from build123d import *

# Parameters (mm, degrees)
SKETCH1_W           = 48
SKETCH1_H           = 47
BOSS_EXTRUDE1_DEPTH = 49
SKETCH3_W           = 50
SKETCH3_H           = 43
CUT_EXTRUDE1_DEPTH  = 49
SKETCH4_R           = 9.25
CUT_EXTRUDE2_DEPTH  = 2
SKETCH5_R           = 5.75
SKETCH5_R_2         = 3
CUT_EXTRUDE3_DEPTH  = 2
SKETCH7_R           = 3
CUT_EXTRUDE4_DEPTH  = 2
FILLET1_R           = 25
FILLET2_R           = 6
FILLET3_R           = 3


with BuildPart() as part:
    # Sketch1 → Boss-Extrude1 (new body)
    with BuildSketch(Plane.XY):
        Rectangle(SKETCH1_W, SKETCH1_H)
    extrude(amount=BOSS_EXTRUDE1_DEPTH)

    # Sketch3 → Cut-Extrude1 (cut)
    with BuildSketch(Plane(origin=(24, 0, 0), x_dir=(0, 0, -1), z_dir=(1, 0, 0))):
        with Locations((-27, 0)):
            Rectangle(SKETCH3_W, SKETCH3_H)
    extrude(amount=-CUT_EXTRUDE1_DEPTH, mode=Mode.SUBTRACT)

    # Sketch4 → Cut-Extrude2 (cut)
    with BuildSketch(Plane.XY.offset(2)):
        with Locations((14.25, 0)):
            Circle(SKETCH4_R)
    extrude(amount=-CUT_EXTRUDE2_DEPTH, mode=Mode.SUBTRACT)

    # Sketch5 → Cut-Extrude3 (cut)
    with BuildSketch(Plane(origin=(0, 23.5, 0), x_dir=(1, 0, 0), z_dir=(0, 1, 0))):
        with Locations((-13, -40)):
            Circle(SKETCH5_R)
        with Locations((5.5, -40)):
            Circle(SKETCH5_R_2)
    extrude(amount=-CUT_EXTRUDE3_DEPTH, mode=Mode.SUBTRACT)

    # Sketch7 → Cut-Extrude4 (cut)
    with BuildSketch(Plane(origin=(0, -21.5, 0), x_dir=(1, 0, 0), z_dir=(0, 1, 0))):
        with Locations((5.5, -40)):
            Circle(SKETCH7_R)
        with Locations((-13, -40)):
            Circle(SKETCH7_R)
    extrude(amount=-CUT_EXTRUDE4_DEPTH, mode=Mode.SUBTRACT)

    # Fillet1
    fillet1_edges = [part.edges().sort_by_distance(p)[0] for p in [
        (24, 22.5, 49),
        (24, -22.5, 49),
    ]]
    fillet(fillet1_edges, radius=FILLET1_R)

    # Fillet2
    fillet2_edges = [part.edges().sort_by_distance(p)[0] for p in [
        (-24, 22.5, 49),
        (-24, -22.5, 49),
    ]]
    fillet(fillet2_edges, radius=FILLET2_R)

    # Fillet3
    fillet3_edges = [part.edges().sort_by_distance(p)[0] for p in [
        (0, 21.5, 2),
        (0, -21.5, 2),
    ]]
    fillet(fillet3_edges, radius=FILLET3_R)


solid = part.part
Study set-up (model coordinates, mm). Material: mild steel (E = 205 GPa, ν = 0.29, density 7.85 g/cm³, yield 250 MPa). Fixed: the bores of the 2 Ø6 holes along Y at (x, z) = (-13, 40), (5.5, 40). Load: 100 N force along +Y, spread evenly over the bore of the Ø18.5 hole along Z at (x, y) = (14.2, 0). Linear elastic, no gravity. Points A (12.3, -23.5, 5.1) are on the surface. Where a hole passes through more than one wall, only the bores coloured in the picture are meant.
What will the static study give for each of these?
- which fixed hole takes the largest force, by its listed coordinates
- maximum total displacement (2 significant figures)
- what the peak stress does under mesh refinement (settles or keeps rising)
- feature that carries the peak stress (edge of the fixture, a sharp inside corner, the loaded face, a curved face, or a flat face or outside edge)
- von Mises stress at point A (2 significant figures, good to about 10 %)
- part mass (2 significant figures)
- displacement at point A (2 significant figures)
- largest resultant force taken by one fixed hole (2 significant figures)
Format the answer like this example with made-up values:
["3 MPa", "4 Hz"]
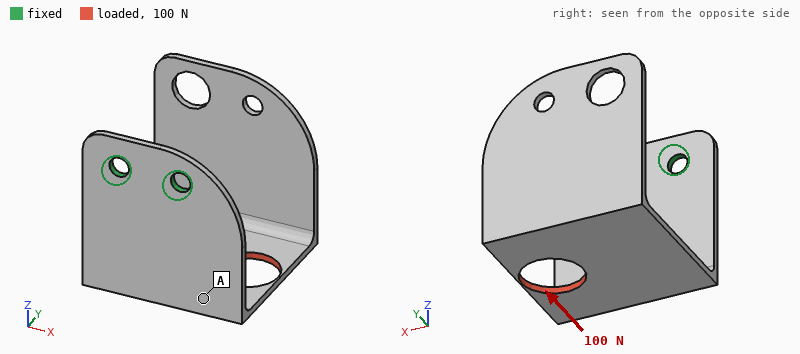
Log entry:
["(5.5, 40)", "0.66 mm", "keeps rising", "edge of the fixture", "19 MPa", "96 g", "0.28 mm", "120 N"]
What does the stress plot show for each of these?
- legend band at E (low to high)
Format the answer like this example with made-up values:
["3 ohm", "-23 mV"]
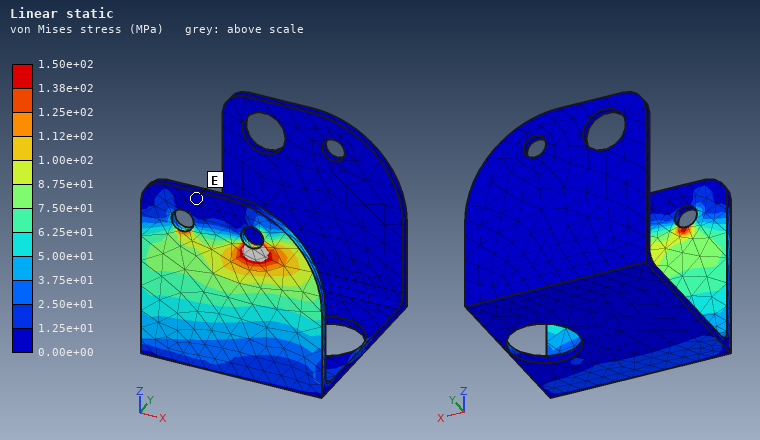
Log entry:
["0.00e+00 to 1.25e+01 MPa"]
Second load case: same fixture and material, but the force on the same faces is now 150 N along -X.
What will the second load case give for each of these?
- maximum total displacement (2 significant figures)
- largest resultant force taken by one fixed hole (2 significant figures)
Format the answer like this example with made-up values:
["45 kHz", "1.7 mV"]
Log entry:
["0.47 mm", "280 N"]
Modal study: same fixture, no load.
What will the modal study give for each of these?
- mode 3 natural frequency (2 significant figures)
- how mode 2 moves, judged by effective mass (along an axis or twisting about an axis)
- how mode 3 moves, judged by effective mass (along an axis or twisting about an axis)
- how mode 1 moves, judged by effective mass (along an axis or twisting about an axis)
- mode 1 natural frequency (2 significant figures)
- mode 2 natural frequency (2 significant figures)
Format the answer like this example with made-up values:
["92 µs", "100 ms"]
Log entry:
["390 Hz", "along X", "along Y", "along Z", "180 Hz", "280 Hz"]
